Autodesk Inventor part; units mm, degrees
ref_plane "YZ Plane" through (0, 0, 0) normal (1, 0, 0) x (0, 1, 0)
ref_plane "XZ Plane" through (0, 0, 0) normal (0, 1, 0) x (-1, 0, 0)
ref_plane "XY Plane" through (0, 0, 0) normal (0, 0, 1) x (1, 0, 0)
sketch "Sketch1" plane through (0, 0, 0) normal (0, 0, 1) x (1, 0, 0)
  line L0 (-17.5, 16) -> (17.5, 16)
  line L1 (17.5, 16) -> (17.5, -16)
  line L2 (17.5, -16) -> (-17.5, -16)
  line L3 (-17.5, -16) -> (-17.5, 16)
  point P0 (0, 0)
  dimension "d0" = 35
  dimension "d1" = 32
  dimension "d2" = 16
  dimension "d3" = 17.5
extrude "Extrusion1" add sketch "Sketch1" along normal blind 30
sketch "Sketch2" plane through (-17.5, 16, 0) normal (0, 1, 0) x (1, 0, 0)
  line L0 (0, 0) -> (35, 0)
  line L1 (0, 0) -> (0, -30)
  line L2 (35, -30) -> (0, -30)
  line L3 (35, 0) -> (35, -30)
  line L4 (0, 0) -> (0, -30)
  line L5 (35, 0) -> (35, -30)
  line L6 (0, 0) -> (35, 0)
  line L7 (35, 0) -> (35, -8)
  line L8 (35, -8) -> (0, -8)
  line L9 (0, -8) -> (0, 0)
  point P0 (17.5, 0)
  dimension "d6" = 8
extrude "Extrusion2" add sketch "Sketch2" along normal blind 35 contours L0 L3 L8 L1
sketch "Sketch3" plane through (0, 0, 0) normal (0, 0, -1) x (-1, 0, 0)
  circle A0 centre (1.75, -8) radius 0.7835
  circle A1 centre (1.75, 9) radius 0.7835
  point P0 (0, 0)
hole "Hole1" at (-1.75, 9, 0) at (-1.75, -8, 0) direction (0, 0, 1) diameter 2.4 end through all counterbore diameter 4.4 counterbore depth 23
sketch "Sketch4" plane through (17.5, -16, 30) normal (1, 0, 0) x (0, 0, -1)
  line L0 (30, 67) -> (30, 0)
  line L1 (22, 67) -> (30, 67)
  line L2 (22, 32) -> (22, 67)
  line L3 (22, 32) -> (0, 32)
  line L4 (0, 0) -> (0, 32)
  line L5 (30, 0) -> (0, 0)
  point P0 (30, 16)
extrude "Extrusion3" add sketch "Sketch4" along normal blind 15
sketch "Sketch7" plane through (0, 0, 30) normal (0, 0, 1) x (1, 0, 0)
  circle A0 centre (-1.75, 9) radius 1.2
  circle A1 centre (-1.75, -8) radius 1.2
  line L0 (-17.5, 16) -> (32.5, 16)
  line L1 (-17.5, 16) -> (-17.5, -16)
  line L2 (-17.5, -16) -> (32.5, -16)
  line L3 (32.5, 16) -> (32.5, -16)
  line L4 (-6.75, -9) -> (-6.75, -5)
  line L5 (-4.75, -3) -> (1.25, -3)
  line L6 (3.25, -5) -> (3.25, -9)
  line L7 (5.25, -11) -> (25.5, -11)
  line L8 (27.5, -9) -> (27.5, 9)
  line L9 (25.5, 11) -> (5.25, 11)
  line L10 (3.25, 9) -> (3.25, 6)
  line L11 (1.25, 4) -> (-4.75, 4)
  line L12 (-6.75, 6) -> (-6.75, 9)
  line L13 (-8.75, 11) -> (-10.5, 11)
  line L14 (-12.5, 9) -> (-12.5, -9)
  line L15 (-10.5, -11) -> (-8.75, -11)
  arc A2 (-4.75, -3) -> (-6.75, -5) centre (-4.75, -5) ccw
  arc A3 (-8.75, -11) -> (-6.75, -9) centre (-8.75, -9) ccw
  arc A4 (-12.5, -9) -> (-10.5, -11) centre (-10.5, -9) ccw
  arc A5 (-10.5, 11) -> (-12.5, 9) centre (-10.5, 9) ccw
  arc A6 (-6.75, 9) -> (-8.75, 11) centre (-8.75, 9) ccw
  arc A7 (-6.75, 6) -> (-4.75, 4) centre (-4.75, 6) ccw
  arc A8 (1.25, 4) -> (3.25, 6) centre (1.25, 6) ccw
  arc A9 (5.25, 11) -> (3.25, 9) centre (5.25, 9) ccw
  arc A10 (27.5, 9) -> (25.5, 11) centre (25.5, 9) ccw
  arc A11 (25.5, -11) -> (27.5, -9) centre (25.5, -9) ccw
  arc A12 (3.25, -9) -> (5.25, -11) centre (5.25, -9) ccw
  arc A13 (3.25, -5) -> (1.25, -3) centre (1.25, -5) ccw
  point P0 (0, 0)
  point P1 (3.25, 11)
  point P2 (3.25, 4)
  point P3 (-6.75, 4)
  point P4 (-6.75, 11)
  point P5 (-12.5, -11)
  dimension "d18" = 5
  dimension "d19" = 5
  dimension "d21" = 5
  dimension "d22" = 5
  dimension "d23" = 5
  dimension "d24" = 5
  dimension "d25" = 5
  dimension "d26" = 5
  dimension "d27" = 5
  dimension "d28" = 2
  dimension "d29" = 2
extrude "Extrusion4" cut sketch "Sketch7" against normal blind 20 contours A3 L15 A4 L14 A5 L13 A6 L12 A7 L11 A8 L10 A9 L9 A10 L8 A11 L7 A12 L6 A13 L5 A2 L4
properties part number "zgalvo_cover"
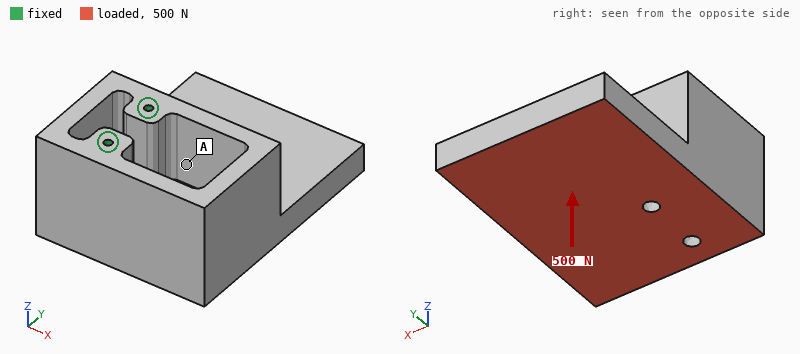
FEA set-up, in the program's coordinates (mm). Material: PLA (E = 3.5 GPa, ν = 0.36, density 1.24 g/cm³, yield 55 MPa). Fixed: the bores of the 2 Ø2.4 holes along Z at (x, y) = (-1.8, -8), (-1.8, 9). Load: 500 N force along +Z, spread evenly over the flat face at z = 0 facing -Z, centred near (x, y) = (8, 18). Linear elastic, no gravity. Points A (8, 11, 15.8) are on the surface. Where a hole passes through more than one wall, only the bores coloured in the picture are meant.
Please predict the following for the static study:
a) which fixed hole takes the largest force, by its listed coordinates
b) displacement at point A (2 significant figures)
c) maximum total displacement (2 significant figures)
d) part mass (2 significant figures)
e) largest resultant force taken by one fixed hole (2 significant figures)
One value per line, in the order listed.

(-1.8, 9)
0.15 mm
0.83 mm
58 g
640 N
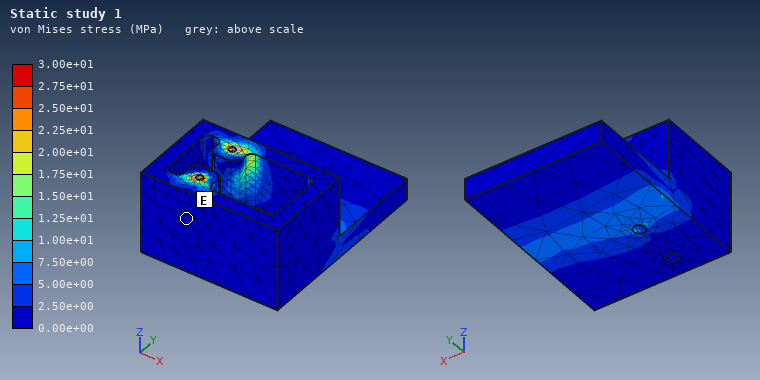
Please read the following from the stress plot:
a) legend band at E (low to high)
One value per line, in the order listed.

0.00e+00 to 2.50e+00 MPa
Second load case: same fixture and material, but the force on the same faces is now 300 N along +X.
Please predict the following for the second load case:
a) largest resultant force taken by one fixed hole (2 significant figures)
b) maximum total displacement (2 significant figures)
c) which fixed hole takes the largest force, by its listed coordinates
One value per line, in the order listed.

350 N
0.86 mm
(-1.8, 9)
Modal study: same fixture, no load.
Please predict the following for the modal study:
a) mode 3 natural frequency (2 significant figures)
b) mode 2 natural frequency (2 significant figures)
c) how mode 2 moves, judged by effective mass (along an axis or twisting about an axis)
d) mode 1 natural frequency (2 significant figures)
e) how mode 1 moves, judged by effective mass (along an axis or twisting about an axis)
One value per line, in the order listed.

1100 Hz
850 Hz
along Y
580 Hz
along X
